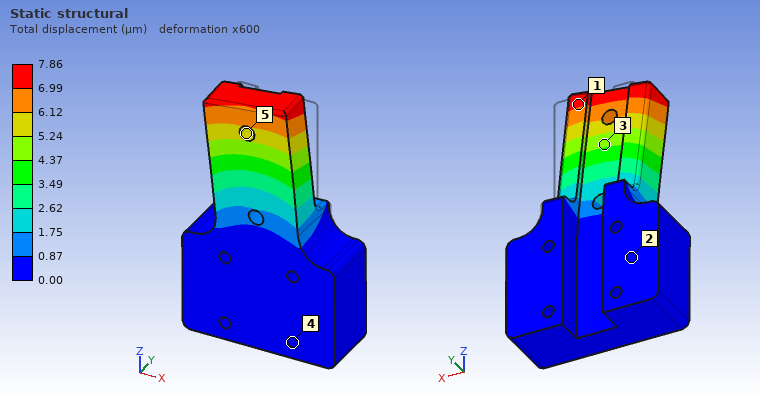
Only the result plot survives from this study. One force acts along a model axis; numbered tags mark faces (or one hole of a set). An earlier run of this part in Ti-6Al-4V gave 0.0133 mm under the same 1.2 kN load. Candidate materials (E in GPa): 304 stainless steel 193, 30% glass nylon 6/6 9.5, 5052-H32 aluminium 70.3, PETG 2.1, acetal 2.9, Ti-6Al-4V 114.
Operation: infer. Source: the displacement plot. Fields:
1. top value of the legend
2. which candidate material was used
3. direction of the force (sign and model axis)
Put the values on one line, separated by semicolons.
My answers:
7.86 µm; 304 stainless steel; -X
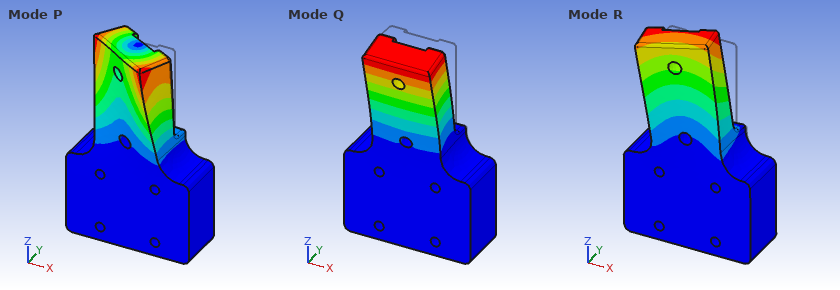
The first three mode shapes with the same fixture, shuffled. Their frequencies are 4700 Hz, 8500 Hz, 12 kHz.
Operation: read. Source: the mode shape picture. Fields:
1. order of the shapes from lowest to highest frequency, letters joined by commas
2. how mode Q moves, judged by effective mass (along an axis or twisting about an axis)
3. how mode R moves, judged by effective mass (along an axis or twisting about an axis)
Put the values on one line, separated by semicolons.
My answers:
Q, R, P; along Y; along X
